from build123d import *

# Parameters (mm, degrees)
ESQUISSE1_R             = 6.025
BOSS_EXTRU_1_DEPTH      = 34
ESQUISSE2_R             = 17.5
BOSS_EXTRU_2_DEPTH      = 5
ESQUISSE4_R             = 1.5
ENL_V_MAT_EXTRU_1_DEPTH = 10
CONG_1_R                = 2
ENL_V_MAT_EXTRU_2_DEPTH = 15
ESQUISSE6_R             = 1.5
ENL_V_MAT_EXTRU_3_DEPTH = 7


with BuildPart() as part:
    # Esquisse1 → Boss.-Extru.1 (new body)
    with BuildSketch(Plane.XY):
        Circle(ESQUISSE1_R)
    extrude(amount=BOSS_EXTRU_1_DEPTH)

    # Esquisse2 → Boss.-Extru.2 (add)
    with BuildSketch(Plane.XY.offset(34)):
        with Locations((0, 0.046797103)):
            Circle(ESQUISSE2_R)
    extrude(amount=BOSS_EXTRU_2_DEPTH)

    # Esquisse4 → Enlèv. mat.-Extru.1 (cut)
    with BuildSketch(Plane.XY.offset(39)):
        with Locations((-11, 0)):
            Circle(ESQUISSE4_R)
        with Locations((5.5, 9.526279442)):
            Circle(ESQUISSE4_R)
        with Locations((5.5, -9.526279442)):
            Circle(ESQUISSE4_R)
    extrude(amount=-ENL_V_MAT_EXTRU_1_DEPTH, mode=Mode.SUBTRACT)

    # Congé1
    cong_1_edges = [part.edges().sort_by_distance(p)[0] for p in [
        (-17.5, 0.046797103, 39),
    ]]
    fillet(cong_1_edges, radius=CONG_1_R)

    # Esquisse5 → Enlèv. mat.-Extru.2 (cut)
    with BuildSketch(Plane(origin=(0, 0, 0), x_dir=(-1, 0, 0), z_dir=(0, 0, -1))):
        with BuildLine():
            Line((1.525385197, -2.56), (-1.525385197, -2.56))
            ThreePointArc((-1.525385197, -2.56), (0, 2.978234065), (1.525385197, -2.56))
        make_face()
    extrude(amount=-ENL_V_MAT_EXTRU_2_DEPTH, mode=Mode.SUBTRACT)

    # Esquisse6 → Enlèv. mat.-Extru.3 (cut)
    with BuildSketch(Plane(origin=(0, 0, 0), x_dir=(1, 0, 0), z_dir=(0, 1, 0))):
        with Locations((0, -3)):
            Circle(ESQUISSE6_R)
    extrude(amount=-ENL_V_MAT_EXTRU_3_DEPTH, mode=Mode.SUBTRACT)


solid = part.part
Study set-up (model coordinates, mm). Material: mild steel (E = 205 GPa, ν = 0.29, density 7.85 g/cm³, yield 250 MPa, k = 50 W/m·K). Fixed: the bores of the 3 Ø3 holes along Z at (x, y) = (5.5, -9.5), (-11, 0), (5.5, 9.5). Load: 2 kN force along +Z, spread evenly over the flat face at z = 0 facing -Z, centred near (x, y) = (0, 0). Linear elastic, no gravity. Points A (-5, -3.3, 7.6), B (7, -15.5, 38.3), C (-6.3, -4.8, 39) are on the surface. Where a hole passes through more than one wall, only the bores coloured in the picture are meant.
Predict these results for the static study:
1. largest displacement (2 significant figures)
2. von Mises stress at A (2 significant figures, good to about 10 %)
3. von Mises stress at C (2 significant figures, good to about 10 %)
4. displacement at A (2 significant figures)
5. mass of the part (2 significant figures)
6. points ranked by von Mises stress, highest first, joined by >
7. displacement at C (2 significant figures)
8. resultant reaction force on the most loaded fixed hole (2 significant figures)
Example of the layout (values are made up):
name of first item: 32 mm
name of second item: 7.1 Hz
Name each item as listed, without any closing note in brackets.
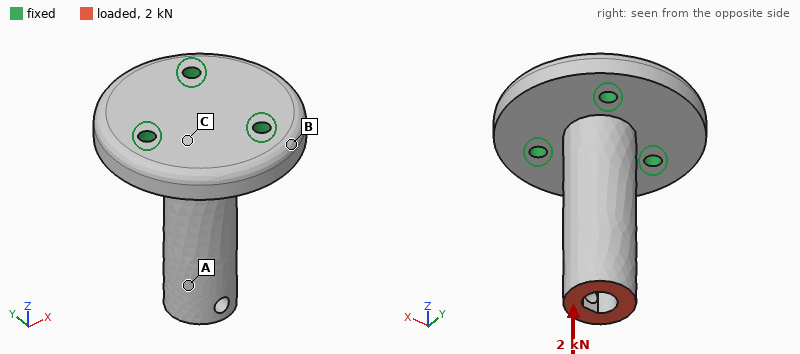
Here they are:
largest displacement: 6.1 µm
von Mises stress at A: 27 MPa
von Mises stress at C: 14 MPa
displacement at A: 4.3 µm
mass of the part: 63 g
points ranked by von Mises stress, highest first, joined by >: A > C > B
displacement at C: 1.2 µm
resultant reaction force on the most loaded fixed hole: 680 N
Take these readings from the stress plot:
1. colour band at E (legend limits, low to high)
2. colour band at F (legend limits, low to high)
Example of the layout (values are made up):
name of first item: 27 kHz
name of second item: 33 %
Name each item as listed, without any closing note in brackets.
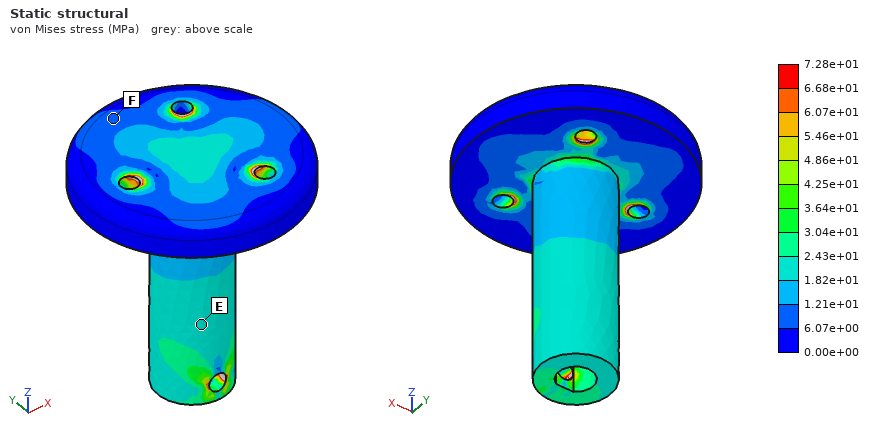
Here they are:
colour band at E: 1.82e+01 to 2.43e+01 MPa
colour band at F: 6.07e+00 to 1.21e+01 MPa
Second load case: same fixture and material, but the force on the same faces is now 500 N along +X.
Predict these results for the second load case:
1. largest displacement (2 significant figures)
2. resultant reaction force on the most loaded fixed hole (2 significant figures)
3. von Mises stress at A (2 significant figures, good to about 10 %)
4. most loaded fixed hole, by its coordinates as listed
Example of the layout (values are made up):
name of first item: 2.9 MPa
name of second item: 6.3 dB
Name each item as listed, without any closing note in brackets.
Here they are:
largest displacement: 51 µm
resultant reaction force on the most loaded fixed hole: 1.1 kN
von Mises stress at A: 21 MPa
most loaded fixed hole, by its coordinates as listed: (-11, 0)
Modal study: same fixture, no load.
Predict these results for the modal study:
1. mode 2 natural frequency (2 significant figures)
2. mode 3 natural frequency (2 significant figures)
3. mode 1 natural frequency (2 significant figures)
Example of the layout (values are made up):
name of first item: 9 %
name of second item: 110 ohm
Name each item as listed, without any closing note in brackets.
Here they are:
mode 2 natural frequency: 6100 Hz
mode 3 natural frequency: 23 kHz
mode 1 natural frequency: 6100 Hz
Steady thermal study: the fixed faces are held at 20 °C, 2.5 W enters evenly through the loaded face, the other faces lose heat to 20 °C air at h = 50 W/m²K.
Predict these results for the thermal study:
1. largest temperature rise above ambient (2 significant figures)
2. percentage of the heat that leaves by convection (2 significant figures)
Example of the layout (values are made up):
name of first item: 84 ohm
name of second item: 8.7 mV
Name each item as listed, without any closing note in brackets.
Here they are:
largest temperature rise above ambient: 17 K
percentage of the heat that leaves by convection: 30 %
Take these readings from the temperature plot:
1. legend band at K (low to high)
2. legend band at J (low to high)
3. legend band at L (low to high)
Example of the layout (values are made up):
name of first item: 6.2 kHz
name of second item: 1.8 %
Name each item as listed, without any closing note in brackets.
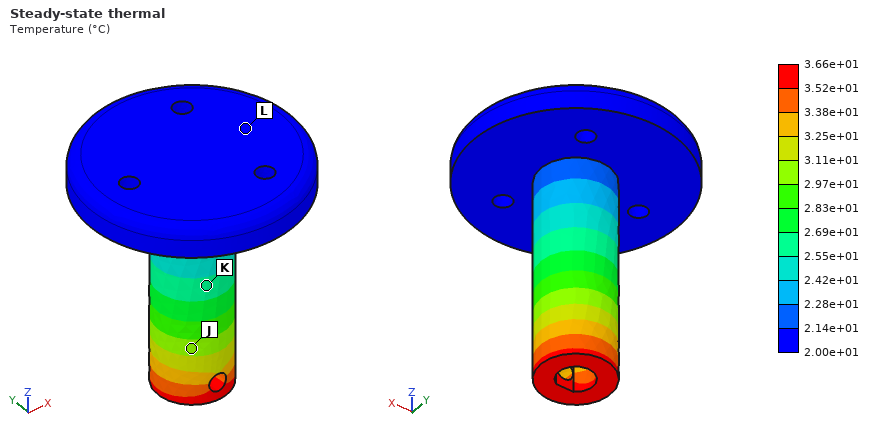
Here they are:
legend band at K: 2.55e+01 to 2.69e+01 °C
legend band at J: 2.97e+01 to 3.11e+01 °C
legend band at L: 2.00e+01 to 2.14e+01 °C
